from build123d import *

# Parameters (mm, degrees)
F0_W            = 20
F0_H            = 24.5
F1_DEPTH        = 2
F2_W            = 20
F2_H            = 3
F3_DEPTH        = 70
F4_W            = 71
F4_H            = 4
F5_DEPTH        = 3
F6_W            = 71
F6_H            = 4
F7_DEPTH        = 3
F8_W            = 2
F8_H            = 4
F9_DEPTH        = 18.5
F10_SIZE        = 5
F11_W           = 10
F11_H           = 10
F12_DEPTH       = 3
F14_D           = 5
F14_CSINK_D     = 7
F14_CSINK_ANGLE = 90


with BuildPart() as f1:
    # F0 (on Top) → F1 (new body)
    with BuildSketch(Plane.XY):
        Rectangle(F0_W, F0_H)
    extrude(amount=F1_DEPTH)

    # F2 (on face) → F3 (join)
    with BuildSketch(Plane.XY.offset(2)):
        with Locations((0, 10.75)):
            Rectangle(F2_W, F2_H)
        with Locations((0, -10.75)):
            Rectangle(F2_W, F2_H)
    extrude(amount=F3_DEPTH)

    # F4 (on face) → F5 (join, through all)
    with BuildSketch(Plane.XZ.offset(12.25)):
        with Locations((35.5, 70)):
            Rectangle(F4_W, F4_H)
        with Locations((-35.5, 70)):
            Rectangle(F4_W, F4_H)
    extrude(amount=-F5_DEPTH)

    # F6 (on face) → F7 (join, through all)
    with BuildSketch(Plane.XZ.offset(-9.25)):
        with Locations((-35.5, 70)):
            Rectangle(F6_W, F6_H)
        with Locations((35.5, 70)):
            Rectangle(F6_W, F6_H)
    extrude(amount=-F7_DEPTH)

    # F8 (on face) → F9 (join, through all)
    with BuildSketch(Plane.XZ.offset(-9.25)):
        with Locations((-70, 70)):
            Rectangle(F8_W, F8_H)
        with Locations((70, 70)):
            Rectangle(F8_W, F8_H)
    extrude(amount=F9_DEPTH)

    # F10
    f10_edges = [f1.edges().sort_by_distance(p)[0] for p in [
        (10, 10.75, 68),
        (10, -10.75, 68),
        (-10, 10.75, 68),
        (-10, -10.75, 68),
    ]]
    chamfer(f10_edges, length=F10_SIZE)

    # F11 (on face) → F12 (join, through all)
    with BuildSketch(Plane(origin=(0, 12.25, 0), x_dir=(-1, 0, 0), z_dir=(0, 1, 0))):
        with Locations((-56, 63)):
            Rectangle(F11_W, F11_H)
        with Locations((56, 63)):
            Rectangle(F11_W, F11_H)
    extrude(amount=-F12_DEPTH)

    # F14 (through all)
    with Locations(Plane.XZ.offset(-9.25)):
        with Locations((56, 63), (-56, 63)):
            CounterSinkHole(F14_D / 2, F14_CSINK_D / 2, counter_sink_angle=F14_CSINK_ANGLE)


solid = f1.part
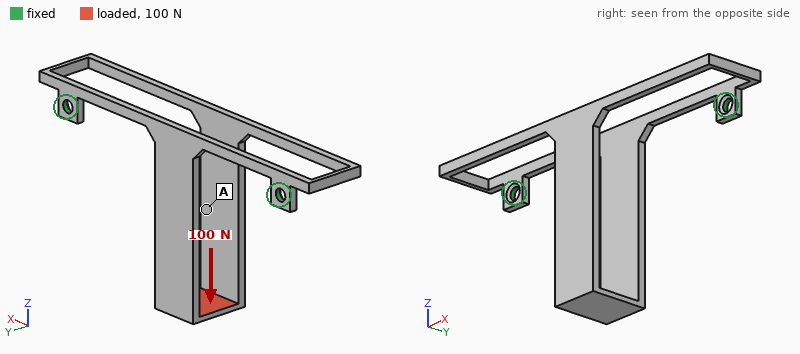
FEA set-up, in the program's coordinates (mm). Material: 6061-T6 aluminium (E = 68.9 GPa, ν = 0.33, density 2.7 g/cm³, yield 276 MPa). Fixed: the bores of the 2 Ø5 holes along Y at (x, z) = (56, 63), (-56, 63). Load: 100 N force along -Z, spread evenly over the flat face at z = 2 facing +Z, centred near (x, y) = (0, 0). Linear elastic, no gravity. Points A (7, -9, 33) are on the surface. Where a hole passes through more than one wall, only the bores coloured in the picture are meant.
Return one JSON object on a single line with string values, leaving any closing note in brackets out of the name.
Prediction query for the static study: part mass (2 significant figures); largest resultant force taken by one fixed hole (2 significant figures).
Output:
{"part mass": "36 g", "largest resultant force taken by one fixed hole": "50 N"}
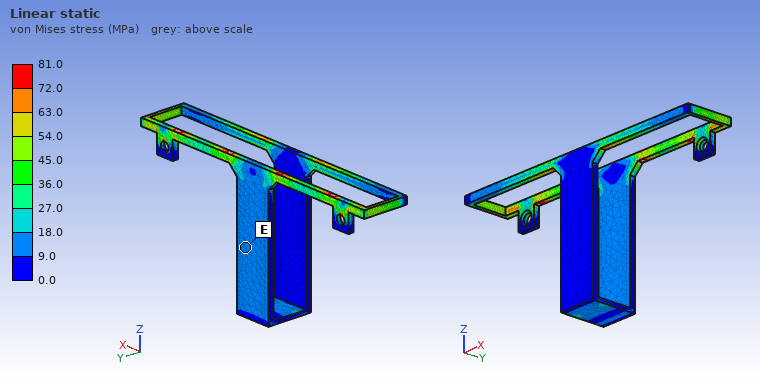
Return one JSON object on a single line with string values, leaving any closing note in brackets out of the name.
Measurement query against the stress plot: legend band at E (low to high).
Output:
{"legend band at E": "9.0 to 18.0 MPa"}
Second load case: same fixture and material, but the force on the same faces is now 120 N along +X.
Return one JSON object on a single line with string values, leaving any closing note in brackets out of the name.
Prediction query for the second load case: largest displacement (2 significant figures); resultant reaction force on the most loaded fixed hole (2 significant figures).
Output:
{"largest displacement": "1.2 mm", "resultant reaction force on the most loaded fixed hole": "110 N"}
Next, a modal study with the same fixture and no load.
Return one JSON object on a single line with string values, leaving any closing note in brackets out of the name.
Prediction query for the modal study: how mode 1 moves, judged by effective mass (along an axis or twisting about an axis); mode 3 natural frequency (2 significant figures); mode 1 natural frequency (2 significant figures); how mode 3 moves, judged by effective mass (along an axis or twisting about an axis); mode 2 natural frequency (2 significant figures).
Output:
{"how mode 1 moves, judged by effective mass": "along Y", "mode 3 natural frequency": "490 Hz", "mode 1 natural frequency": "140 Hz", "how mode 3 moves, judged by effective mass": "along X", "mode 2 natural frequency": "410 Hz"}
